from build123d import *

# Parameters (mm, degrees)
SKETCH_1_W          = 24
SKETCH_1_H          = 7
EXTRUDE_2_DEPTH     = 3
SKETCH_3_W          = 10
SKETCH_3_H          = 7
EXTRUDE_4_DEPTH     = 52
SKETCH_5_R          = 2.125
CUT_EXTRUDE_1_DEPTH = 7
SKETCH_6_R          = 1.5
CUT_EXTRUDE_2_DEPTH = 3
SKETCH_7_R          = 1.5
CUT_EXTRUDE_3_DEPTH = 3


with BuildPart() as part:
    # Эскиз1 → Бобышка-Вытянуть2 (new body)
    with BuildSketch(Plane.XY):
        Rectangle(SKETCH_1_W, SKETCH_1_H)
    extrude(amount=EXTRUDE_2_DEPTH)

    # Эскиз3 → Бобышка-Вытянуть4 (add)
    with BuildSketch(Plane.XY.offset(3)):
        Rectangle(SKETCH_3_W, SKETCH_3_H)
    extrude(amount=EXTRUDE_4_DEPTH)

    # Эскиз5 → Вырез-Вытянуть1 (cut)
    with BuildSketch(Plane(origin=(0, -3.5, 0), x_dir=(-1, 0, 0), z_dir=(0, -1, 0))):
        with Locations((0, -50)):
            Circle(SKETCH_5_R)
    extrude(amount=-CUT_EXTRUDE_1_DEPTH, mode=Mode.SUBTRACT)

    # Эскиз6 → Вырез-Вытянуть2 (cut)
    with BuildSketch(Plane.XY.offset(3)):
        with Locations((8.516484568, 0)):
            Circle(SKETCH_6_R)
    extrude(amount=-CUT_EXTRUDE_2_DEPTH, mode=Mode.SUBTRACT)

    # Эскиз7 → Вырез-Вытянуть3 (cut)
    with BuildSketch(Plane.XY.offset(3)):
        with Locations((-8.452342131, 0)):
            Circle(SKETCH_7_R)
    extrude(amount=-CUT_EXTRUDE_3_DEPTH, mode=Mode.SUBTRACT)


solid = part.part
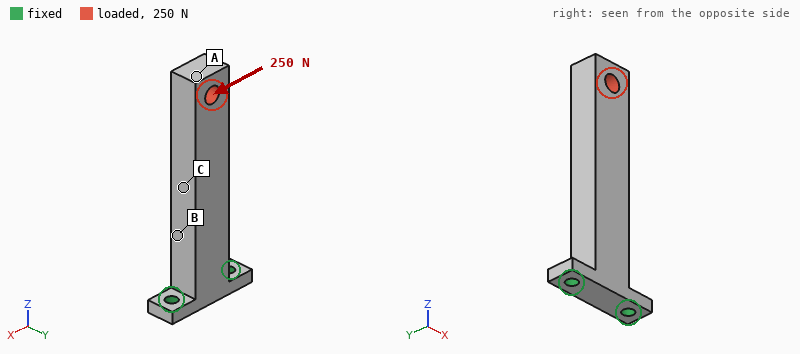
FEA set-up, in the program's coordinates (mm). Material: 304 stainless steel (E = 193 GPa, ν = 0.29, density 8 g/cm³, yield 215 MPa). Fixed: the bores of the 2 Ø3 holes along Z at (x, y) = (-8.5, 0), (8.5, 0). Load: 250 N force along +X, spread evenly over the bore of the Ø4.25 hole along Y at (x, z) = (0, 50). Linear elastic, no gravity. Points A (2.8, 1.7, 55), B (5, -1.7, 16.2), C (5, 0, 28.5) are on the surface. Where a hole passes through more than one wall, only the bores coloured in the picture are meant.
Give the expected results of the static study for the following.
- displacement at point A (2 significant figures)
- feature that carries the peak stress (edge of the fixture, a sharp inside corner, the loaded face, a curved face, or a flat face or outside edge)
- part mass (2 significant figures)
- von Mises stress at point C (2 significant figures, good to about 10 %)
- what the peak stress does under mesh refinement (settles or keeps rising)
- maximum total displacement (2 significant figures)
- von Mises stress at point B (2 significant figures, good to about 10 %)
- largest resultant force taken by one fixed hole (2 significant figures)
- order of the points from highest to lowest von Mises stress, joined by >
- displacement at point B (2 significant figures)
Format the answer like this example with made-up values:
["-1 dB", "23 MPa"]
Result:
["0.13 mm", "edge of the fixture", "32 g", "46 MPa", "keeps rising", "0.13 mm", "72 MPa", "980 N", "B > C > A", "0.022 mm"]
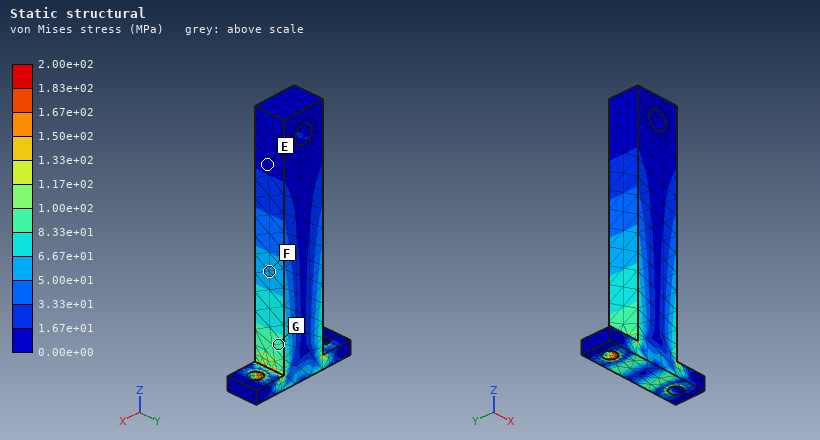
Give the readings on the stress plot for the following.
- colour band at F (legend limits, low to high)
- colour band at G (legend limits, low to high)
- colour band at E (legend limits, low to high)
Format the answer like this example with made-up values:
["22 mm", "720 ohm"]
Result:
["5.00e+01 to 6.67e+01 MPa", "8.33e+01 to 1.00e+02 MPa", "0.00e+00 to 1.67e+01 MPa"]
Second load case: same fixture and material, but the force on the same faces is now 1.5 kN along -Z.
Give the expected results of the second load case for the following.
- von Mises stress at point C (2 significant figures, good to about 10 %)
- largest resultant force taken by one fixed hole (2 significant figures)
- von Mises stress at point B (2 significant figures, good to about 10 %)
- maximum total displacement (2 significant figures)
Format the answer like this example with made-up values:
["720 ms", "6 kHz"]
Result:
["21 MPa", "800 N", "21 MPa", "9.7 µm"]
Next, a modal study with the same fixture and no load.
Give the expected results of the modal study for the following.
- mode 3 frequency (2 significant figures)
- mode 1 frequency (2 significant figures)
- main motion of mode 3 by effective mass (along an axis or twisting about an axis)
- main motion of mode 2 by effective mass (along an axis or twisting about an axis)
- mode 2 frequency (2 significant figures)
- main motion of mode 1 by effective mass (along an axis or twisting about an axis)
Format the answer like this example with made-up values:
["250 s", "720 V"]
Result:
["9000 Hz", "1200 Hz", "along Y", "along X", "2400 Hz", "along Y"]
